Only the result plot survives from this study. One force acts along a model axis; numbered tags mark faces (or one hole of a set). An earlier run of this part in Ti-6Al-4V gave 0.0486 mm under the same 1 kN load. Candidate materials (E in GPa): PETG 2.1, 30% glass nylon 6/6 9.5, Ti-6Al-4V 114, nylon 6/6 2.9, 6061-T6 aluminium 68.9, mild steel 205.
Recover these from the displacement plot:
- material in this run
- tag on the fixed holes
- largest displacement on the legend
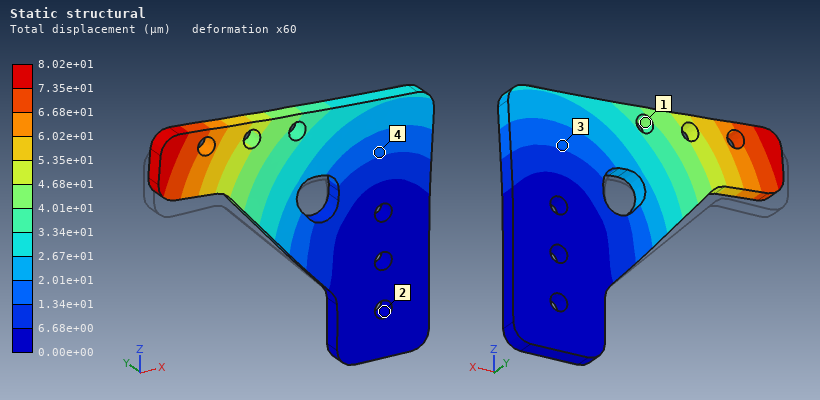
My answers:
6061-T6 aluminium
2
8.02e+01 µm
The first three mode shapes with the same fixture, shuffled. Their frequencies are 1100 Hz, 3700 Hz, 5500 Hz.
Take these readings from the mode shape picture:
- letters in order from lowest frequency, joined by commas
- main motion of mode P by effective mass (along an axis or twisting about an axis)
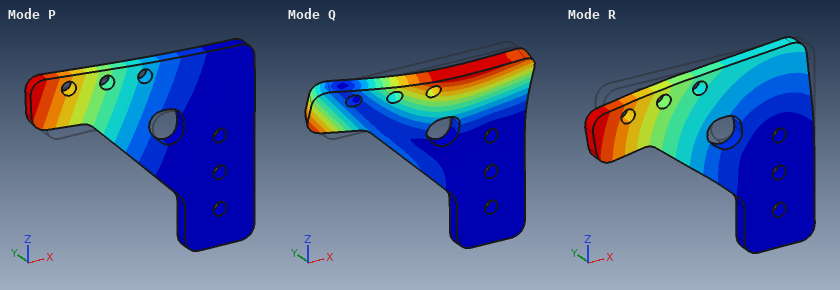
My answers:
P, Q, R
along Y
